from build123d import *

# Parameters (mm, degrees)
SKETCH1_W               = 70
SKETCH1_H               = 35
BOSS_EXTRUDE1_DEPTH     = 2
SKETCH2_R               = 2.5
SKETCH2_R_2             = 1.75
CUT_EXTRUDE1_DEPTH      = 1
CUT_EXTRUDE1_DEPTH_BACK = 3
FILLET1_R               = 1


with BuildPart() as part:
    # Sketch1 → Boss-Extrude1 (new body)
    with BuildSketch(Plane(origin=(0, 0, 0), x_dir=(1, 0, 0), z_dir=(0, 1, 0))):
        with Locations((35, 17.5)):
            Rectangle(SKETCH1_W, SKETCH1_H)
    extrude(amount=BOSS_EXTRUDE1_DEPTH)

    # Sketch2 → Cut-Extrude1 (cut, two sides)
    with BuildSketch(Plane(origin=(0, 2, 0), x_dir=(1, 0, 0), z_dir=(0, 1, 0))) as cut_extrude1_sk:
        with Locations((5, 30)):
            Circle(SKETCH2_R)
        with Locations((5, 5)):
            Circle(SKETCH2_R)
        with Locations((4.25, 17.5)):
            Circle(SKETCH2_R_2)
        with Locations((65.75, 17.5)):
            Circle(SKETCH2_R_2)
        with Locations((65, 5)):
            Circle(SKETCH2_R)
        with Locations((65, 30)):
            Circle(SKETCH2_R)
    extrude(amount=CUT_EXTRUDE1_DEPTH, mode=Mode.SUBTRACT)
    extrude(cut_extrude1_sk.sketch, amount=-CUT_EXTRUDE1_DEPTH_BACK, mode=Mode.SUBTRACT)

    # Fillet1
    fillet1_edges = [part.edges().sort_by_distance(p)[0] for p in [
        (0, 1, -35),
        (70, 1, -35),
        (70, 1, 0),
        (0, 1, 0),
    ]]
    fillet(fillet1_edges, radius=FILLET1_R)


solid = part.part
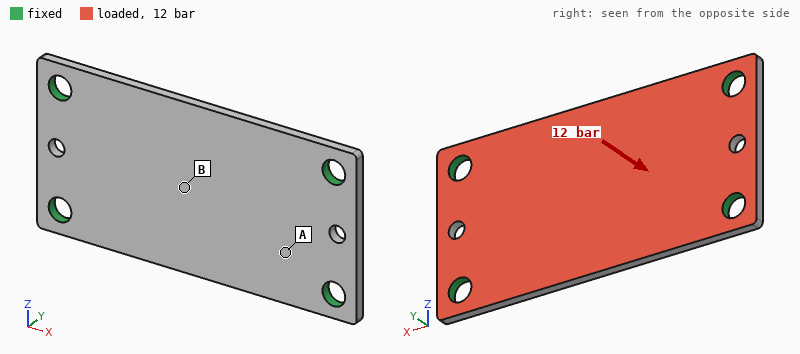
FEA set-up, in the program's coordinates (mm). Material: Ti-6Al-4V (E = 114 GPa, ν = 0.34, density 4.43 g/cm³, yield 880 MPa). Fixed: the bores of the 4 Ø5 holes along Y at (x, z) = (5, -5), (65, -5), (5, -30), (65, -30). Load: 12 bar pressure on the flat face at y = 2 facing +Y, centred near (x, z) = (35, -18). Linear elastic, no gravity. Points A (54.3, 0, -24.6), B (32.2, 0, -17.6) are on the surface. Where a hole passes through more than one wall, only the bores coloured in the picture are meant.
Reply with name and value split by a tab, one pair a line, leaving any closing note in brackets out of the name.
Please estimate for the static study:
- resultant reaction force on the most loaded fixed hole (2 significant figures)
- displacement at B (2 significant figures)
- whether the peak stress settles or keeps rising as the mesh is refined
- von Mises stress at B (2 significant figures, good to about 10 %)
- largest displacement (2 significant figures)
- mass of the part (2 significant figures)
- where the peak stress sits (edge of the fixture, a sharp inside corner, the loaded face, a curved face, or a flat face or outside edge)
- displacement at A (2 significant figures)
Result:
resultant reaction force on the most loaded fixed hole	710 N
displacement at B	0.44 mm
whether the peak stress settles or keeps rising as the mesh is refined	keeps rising
von Mises stress at B	210 MPa
largest displacement	0.48 mm
mass of the part	21 g
where the peak stress sits	edge of the fixture
displacement at A	0.16 mm
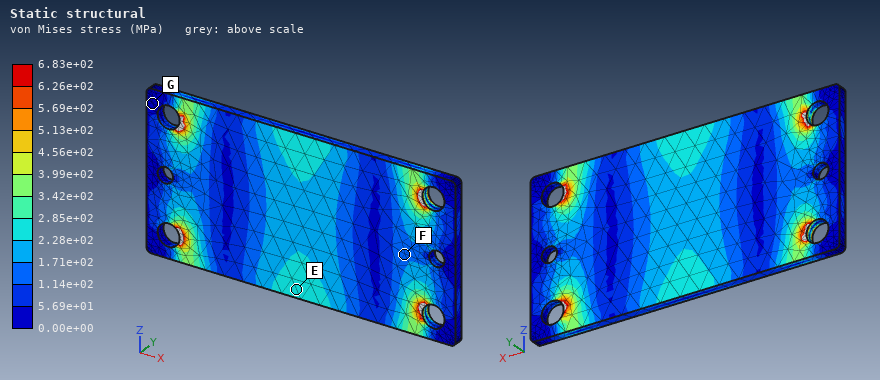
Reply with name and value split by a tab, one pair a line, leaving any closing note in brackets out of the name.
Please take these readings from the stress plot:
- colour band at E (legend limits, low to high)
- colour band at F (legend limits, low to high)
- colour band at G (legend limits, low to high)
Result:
colour band at E	2.28e+02 to 2.85e+02 MPa
colour band at F	1.14e+02 to 1.71e+02 MPa
colour band at G	0.00e+00 to 5.69e+01 MPa
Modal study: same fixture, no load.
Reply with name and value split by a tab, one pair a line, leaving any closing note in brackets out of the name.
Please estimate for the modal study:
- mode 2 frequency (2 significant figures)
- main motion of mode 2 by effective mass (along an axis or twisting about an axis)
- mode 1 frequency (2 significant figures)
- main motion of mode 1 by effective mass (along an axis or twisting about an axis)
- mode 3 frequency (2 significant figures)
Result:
mode 2 frequency	4700 Hz
main motion of mode 2 by effective mass	twisting about X
mode 1 frequency	3100 Hz
main motion of mode 1 by effective mass	along Y
mode 3 frequency	8400 Hz
